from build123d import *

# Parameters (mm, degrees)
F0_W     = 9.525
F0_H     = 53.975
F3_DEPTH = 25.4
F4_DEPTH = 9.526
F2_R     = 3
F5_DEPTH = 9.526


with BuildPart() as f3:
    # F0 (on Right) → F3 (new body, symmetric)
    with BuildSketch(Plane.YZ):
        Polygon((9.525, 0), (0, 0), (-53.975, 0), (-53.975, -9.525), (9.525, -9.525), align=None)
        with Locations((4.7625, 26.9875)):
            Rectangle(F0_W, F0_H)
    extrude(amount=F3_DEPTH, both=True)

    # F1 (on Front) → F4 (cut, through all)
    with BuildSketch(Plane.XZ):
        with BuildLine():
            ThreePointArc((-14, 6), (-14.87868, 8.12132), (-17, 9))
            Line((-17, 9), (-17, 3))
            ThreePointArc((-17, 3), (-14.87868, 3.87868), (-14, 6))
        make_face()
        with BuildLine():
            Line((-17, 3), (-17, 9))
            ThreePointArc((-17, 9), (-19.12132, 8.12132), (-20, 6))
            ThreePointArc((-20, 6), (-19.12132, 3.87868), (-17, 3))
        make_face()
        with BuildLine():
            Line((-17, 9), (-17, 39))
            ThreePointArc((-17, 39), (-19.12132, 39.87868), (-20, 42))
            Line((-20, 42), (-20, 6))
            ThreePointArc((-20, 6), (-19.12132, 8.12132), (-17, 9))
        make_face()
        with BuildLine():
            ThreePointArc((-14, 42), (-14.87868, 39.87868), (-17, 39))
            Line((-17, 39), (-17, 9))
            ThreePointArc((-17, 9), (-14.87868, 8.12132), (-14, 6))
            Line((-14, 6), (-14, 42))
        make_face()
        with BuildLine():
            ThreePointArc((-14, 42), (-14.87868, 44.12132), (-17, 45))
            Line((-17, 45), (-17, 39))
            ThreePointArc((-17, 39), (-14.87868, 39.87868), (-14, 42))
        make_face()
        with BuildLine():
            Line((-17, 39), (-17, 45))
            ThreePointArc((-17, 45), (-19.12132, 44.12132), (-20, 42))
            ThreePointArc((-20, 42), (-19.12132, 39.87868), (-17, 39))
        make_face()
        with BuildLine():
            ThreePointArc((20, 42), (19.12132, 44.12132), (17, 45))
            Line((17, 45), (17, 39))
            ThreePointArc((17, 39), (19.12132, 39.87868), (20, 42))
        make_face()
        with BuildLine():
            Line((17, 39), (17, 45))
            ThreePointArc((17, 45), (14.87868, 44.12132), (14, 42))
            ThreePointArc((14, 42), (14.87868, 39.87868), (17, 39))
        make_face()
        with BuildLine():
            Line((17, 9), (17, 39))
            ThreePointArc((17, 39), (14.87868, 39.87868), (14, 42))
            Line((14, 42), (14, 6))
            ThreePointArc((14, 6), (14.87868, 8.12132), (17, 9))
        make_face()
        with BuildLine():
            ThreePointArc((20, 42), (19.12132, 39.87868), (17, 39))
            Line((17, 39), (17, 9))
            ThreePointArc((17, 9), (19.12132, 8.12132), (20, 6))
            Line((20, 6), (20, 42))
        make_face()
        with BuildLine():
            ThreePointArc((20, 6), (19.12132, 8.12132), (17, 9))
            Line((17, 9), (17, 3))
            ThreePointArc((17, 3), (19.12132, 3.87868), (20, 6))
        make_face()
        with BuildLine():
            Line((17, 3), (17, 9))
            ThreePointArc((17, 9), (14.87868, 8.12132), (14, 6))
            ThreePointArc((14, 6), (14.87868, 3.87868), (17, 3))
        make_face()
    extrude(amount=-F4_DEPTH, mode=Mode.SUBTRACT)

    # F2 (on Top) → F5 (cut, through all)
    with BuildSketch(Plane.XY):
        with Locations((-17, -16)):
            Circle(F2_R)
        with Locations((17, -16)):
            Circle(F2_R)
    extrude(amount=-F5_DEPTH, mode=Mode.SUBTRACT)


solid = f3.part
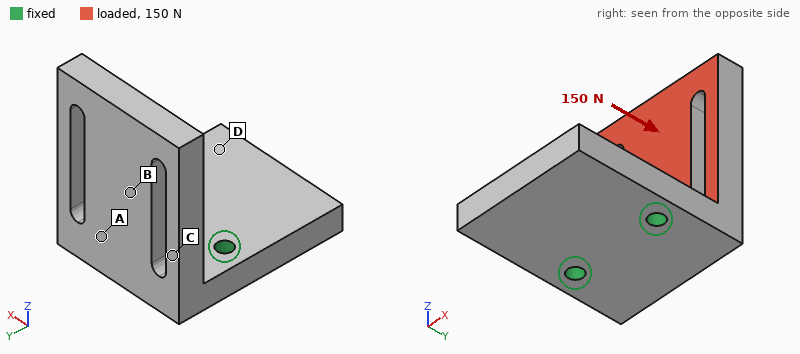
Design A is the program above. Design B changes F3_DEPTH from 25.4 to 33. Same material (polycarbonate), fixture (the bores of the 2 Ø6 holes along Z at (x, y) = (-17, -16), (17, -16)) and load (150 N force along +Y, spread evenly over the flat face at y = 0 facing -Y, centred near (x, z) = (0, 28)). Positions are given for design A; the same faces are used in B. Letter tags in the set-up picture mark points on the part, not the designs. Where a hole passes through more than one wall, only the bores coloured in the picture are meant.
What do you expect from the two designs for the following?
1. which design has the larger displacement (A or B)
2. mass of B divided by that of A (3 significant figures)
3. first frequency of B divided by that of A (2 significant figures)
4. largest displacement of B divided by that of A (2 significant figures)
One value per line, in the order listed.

A
1.33
0.98
0.76
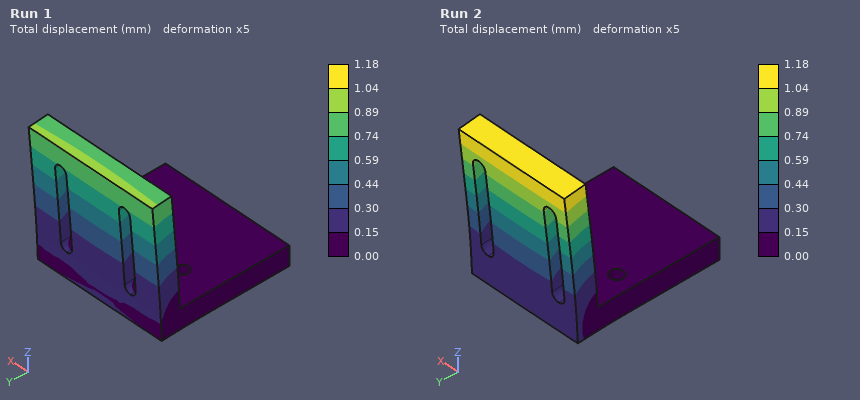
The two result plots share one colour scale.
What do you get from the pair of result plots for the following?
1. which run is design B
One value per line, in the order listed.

Run 1
